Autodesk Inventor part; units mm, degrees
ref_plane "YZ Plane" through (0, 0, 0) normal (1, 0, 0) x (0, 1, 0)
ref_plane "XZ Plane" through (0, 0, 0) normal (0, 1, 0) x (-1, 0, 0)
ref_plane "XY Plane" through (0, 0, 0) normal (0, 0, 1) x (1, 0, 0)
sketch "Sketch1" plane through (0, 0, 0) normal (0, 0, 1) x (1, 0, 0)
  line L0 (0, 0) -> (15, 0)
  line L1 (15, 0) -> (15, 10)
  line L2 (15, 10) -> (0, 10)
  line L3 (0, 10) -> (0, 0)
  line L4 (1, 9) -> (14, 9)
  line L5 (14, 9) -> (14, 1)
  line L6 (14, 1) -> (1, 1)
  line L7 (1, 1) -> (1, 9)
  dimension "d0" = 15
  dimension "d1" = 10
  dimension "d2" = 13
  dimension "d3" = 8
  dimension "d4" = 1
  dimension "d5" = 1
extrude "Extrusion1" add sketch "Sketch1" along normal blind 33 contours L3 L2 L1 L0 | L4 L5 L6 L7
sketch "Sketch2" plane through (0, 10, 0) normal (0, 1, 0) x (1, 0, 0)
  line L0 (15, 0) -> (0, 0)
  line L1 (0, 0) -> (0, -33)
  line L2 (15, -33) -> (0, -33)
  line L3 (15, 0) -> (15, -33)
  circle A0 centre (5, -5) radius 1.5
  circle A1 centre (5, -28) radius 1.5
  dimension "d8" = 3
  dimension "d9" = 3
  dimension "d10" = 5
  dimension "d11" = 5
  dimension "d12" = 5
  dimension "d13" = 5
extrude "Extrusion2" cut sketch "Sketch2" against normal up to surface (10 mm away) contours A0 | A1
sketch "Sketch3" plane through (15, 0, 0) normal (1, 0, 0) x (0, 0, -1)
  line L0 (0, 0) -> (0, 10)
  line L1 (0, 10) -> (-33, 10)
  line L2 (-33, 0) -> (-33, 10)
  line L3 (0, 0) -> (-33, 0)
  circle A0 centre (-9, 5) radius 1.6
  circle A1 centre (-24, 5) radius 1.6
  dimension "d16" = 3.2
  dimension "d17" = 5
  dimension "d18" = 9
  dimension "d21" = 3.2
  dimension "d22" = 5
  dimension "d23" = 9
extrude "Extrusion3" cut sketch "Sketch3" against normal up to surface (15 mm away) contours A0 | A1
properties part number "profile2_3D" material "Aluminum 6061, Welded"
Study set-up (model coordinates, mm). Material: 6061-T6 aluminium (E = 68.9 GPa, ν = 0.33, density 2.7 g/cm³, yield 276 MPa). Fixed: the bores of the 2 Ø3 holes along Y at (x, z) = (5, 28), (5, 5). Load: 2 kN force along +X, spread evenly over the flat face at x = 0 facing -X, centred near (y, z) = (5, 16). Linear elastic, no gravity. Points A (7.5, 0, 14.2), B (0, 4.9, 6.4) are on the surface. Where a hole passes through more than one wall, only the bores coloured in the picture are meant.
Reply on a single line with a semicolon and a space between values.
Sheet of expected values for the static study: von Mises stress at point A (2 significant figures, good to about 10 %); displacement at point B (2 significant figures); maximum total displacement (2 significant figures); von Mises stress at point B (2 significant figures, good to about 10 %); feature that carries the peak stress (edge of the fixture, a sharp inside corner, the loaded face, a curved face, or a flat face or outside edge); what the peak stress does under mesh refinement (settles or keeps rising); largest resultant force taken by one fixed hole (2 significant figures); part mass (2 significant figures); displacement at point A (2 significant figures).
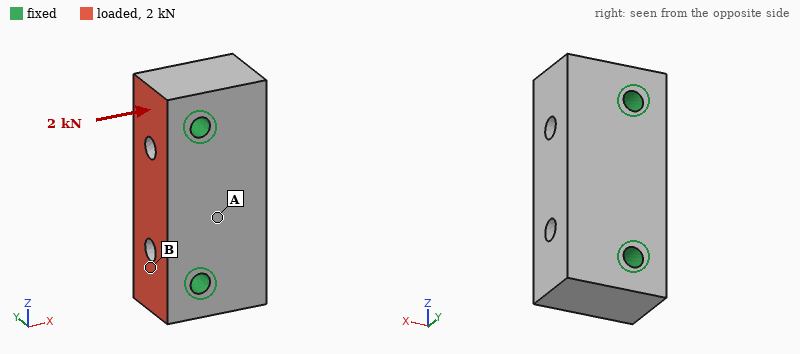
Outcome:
4.6 MPa; 0.70 µm; 2.4 µm; 11 MPa; edge of the fixture; keeps rising; 1.0 kN; 12 g; 1.9 µm
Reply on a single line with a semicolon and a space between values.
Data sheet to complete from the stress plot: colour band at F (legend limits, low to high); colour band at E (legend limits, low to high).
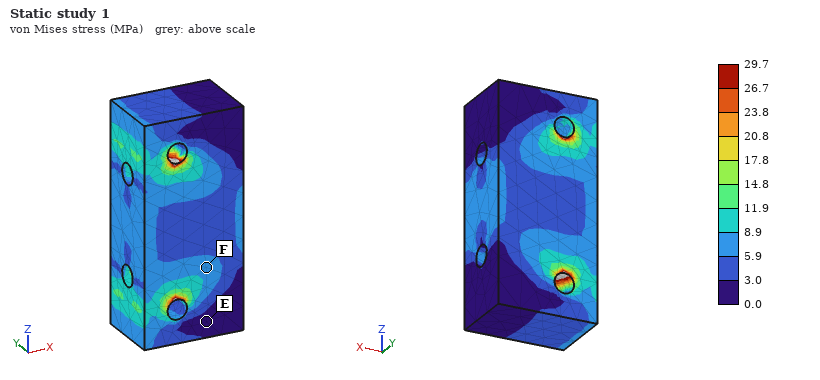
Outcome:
5.9 to 8.9 MPa; 0.0 to 3.0 MPa
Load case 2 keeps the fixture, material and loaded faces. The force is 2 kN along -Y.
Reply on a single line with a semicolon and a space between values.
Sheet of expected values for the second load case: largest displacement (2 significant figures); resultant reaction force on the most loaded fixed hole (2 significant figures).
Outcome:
8.1 µm; 1.0 kN
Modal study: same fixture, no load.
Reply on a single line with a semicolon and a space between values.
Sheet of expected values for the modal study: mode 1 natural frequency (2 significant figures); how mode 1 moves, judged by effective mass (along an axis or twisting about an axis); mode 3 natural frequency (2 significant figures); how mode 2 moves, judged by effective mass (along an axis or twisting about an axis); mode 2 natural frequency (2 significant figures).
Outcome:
35 kHz; along Y; 49 kHz; along X; 46 kHz
